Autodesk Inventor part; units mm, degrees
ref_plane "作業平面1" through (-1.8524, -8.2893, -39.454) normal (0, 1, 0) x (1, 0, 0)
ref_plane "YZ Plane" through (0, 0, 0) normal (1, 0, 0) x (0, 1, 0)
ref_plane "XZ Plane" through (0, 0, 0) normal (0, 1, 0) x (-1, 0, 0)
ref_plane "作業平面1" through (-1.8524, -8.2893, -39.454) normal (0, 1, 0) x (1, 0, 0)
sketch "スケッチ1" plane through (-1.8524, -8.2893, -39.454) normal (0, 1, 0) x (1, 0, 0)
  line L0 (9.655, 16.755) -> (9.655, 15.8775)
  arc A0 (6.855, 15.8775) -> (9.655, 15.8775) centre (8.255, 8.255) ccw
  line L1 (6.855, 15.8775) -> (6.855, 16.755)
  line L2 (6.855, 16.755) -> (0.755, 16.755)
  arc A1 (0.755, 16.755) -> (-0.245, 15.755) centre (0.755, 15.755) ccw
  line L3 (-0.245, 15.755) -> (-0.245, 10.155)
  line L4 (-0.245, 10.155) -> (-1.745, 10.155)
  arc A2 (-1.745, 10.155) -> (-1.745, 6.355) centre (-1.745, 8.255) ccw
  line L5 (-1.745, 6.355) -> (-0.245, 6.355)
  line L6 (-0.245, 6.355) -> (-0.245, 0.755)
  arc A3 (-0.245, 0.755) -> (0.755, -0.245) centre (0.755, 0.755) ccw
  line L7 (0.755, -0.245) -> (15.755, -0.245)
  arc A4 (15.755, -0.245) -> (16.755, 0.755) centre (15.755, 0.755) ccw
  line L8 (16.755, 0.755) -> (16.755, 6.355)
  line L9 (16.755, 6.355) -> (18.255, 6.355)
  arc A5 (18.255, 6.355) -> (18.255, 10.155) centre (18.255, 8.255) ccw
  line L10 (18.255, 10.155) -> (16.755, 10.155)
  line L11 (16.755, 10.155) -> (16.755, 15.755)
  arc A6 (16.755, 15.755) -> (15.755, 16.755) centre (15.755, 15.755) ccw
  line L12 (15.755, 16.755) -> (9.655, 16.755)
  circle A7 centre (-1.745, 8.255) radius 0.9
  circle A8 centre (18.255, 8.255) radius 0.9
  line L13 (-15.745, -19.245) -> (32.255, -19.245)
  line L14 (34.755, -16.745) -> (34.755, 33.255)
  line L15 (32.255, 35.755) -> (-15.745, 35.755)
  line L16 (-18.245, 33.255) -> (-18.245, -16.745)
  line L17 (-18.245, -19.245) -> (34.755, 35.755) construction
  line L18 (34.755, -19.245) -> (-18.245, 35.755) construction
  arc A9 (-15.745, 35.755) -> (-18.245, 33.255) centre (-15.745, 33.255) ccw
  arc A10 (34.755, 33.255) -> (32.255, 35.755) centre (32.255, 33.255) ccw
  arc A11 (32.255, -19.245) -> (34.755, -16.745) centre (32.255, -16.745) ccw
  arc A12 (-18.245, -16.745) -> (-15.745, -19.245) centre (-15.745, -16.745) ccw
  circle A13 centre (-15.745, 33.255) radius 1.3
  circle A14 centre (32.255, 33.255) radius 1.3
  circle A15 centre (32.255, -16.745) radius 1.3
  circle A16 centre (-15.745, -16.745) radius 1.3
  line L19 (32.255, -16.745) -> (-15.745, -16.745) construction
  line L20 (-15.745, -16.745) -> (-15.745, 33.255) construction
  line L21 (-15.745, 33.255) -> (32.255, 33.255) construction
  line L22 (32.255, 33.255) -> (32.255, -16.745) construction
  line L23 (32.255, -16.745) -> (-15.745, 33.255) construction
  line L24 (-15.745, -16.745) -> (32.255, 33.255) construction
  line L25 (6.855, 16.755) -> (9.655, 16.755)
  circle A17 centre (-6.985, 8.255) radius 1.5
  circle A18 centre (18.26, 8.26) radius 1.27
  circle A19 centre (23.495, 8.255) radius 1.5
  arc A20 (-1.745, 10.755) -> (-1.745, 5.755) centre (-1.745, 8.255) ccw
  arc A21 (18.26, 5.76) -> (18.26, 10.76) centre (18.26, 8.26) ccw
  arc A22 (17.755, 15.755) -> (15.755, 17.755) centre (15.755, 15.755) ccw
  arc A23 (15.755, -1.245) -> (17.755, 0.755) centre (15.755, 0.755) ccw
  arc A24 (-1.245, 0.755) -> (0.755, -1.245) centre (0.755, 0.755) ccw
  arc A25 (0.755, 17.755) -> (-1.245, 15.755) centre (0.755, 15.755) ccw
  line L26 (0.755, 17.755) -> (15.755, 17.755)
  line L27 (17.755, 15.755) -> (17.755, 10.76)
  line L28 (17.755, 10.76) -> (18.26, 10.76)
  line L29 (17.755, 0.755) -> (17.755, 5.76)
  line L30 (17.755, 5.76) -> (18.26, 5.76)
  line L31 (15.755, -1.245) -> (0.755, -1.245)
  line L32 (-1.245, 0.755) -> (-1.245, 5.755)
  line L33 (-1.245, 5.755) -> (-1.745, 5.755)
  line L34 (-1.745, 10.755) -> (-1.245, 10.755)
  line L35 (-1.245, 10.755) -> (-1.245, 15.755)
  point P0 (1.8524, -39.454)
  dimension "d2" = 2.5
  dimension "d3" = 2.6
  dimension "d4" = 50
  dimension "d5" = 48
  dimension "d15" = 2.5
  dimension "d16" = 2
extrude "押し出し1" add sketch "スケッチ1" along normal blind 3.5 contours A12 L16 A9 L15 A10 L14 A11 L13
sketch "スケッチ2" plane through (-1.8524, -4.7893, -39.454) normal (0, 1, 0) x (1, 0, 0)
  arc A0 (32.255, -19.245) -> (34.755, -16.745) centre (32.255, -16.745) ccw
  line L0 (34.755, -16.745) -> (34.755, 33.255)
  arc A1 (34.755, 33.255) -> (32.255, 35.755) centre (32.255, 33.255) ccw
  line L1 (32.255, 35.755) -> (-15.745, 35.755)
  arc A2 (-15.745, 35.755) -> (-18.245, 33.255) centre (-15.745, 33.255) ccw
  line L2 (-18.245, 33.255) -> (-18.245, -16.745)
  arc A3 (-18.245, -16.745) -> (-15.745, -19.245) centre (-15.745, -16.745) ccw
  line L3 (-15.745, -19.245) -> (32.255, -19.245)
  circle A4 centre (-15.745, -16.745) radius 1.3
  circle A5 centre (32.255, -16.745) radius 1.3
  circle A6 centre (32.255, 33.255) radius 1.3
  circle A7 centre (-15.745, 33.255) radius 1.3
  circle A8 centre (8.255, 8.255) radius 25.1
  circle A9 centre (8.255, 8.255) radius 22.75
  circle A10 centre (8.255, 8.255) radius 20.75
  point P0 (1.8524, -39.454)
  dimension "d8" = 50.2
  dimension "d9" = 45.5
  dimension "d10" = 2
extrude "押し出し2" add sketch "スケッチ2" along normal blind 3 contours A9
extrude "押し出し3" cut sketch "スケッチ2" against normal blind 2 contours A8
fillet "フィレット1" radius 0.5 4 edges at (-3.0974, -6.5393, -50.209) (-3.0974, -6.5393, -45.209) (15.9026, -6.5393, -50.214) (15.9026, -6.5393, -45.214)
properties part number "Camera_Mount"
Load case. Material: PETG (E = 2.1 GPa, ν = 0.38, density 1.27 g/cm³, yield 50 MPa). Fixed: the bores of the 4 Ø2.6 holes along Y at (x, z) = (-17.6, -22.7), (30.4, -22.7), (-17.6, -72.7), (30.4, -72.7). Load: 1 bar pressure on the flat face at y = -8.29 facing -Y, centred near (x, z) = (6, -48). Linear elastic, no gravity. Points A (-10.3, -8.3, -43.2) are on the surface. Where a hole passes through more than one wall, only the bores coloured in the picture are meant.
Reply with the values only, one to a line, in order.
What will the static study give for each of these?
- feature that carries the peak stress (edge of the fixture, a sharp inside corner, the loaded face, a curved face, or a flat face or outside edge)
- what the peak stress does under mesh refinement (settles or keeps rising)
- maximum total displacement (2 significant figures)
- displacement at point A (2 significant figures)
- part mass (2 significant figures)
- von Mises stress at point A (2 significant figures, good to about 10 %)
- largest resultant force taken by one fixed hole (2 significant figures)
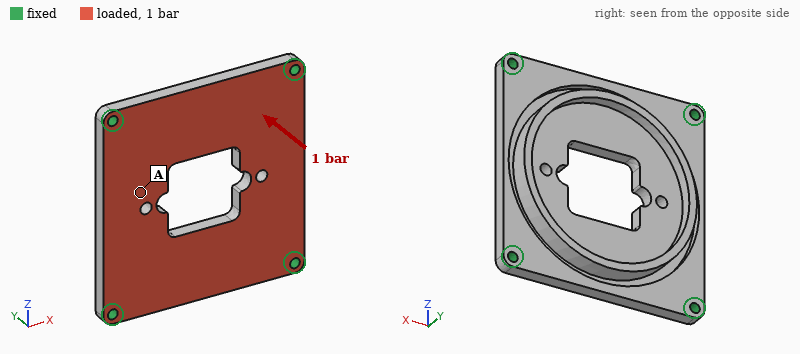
edge of the fixture
keeps rising
0.51 mm
0.40 mm
11 g
4.8 MPa
65 N
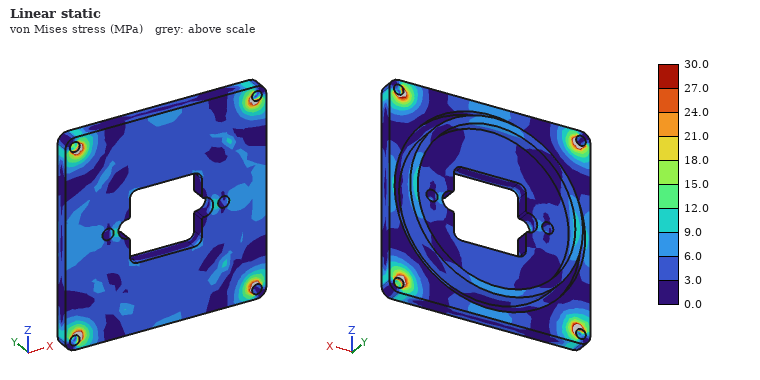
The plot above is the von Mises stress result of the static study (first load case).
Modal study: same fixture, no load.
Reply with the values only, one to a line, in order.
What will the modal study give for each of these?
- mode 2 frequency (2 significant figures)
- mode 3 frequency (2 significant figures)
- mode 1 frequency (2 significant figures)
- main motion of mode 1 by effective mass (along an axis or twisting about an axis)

1800 Hz
1800 Hz
1300 Hz
along Y
